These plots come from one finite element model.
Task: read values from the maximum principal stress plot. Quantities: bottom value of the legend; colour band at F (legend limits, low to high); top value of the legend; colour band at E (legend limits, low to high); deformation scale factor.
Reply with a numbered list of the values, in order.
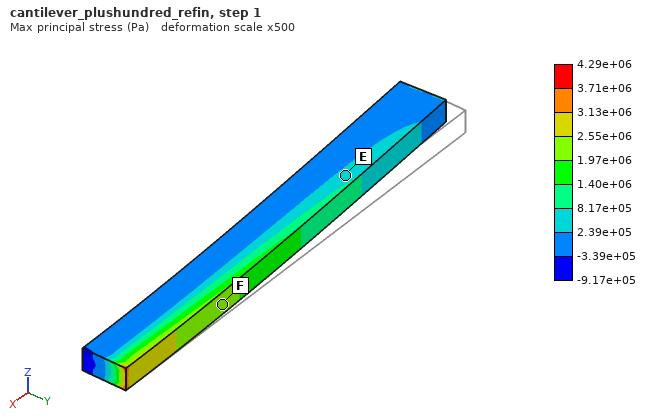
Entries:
1. -9.17e+05 Pa
2. 1.97e+06 to 2.55e+06 Pa
3. 4.29e+06 Pa
4. 2.39e+05 to 8.17e+05 Pa
5. 500
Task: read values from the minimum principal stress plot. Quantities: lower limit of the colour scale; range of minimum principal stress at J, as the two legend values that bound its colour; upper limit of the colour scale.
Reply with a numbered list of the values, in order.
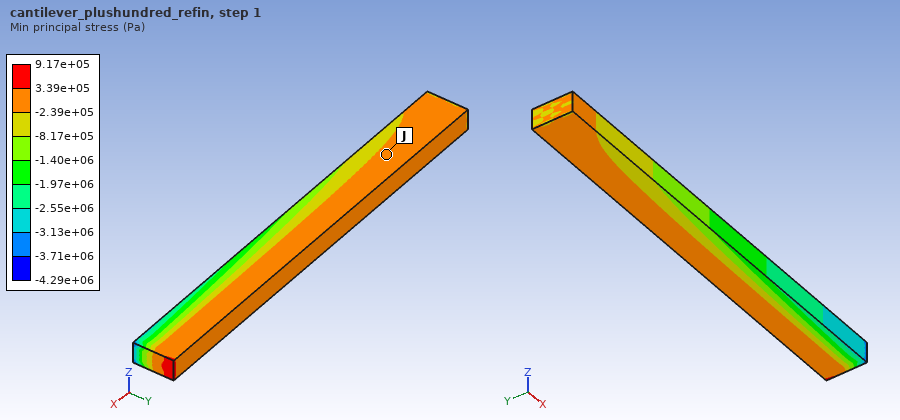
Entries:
1. -4.29e+06 Pa
2. -2.39e+05 to 3.39e+05 Pa
3. 9.17e+05 Pa
